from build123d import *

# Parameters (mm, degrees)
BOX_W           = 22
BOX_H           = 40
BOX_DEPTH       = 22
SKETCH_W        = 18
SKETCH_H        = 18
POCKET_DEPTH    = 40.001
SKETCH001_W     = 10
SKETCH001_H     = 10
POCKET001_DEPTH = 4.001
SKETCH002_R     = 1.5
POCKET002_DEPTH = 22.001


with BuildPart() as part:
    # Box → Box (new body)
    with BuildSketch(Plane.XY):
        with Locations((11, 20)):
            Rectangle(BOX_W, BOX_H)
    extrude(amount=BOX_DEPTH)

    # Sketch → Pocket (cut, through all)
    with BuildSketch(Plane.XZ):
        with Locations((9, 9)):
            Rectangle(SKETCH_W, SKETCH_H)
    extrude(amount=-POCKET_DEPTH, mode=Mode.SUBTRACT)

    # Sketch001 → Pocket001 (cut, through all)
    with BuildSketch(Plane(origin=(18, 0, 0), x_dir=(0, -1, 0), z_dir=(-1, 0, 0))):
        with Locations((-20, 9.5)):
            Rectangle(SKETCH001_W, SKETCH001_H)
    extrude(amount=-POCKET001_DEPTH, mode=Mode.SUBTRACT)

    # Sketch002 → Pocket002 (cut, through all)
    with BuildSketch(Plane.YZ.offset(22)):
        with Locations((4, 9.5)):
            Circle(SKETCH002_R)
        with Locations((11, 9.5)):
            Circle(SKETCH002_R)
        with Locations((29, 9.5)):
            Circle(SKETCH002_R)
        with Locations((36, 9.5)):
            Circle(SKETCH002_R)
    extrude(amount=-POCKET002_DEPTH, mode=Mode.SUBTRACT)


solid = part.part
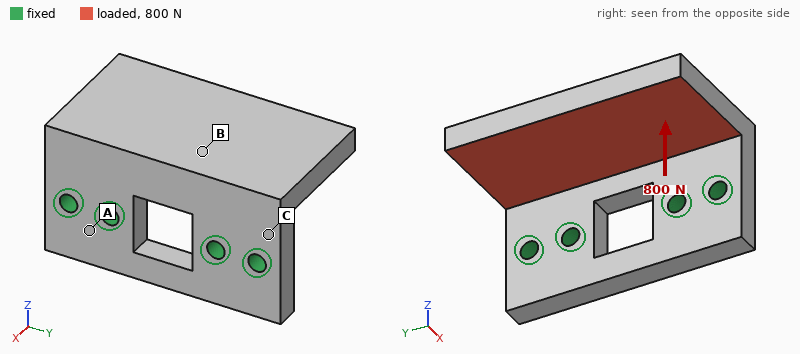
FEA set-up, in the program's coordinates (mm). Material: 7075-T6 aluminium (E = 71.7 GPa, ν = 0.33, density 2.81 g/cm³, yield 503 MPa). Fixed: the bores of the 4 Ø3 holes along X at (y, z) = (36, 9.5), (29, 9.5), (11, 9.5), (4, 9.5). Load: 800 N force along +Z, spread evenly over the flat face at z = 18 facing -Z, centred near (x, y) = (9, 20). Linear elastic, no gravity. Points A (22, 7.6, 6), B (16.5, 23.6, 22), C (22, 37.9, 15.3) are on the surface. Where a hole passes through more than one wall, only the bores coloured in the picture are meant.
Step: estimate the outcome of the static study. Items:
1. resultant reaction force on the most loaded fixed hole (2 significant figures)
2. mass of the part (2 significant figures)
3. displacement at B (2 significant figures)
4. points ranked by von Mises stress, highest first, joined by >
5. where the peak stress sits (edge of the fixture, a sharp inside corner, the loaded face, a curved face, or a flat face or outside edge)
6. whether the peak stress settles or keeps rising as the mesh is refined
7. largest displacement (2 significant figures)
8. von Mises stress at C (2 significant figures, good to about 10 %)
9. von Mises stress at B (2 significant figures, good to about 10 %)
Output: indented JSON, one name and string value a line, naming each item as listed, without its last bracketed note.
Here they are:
{
  "resultant reaction force on the most loaded fixed hole": "270 N",
  "mass of the part": "17 g",
  "displacement at B": "0.058 mm",
  "points ranked by von Mises stress, highest first, joined by >": "C > B > A",
  "where the peak stress sits": "edge of the fixture",
  "whether the peak stress settles or keeps rising as the mesh is refined": "keeps rising",
  "largest displacement": "0.19 mm",
  "von Mises stress at C": "93 MPa",
  "von Mises stress at B": "43 MPa"
}
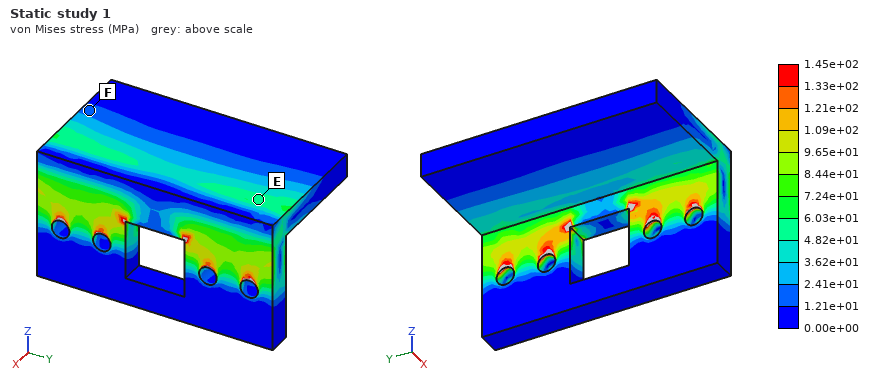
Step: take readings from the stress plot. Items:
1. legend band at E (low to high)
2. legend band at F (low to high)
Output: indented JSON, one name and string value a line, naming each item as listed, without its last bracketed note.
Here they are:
{
  "legend band at E": "4.82e+01 to 6.03e+01 MPa",
  "legend band at F": "1.21e+01 to 2.41e+01 MPa"
}
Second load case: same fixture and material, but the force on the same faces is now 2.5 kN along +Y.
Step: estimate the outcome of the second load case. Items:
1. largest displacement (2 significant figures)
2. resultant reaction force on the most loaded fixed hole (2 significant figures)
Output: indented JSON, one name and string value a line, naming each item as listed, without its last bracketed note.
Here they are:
{
  "largest displacement": "0.12 mm",
  "resultant reaction force on the most loaded fixed hole": "1.2 kN"
}
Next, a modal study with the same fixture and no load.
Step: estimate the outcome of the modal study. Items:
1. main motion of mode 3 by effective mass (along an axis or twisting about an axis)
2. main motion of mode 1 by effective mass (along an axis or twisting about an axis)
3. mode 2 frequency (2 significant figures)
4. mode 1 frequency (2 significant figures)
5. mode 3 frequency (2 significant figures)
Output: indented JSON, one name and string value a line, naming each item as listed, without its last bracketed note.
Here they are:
{
  "main motion of mode 3 by effective mass": "along Y",
  "main motion of mode 1 by effective mass": "along Z",
  "mode 2 frequency": "8200 Hz",
  "mode 1 frequency": "4300 Hz",
  "mode 3 frequency": "13 kHz"
}
